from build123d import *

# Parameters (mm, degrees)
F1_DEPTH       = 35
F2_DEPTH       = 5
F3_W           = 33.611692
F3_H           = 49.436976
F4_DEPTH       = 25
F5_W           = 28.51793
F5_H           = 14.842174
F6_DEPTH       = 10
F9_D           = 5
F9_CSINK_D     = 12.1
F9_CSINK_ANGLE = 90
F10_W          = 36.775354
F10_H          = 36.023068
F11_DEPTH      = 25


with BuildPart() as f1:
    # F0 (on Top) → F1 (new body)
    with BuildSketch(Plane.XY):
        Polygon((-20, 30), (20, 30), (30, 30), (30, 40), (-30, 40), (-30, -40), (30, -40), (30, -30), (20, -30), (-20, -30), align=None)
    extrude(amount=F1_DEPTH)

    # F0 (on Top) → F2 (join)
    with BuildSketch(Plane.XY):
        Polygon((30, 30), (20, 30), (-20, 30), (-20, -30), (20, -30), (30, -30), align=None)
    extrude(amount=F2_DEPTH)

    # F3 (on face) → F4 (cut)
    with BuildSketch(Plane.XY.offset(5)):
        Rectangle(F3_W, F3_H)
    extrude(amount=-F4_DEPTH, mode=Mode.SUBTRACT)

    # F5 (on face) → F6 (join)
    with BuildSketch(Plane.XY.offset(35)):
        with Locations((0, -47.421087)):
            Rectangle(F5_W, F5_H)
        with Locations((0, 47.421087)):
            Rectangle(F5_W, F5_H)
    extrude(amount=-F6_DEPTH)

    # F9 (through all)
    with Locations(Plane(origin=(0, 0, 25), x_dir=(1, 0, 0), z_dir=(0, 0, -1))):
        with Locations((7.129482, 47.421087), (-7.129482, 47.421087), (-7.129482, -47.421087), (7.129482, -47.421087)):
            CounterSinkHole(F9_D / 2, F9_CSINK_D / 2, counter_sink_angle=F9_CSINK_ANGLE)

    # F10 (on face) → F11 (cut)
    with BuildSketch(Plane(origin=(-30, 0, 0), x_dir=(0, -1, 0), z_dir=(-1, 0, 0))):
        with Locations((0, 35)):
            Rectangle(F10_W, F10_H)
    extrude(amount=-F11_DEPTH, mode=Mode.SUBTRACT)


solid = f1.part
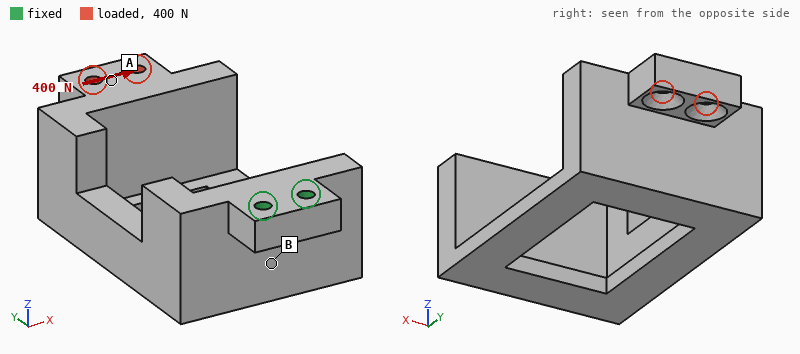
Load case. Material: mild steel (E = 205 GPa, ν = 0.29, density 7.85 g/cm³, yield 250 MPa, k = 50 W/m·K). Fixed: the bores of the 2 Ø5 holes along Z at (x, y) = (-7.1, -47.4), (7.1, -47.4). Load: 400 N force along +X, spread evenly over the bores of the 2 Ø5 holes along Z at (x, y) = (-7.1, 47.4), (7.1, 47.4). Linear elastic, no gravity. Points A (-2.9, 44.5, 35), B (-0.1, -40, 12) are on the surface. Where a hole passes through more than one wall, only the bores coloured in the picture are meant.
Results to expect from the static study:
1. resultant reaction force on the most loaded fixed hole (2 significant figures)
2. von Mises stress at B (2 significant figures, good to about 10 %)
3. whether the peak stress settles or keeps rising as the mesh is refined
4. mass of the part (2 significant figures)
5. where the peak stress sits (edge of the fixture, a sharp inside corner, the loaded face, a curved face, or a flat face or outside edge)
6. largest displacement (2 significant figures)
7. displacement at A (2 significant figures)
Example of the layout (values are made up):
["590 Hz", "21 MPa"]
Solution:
["2.1 kN", "28 MPa", "keeps rising", "550 g", "edge of the fixture", "0.13 mm", "0.12 mm"]
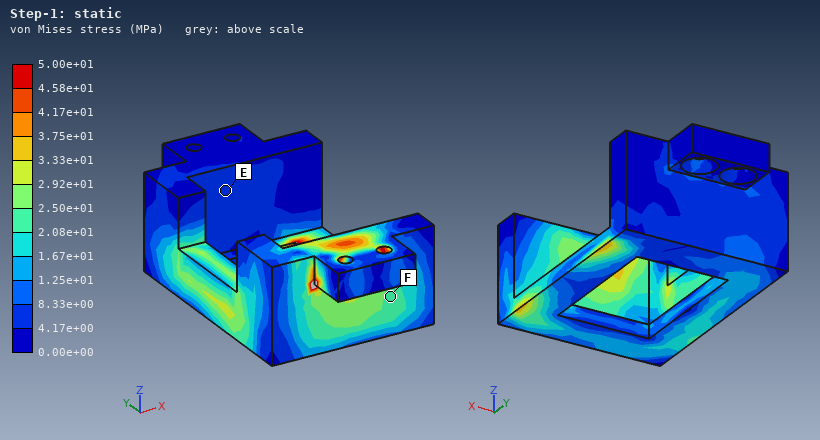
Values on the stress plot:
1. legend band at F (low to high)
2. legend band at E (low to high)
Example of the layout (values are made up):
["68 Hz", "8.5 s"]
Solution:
["2.08e+01 to 2.50e+01 MPa", "4.17e+00 to 8.33e+00 MPa"]
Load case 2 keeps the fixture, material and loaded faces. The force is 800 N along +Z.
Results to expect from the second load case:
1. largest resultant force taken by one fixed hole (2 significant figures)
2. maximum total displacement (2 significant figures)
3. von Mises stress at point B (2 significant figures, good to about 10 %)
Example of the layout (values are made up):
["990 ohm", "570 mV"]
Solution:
["700 N", "0.57 mm", "38 MPa"]
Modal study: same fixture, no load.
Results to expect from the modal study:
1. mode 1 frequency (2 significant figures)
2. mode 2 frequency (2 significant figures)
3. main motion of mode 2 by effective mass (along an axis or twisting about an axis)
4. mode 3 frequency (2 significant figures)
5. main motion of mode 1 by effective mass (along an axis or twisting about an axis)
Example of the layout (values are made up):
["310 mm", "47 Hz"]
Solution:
["470 Hz", "730 Hz", "along X", "1500 Hz", "along Z"]
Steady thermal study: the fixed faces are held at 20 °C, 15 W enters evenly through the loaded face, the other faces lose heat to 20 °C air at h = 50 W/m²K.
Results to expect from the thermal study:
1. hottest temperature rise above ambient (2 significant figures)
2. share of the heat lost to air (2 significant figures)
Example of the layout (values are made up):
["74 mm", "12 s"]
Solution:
["42 K", "88 %"]
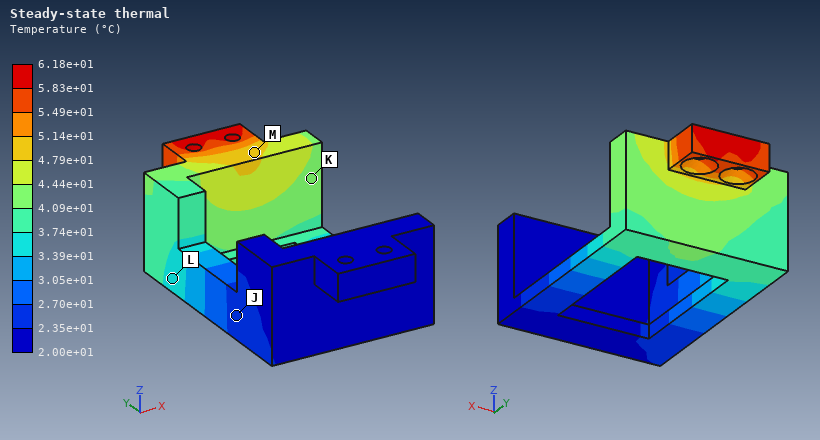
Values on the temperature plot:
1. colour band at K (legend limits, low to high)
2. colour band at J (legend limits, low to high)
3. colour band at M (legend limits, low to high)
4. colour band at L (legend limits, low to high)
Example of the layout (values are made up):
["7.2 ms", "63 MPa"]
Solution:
["4.09e+01 to 4.44e+01 °C", "2.35e+01 to 2.70e+01 °C", "4.79e+01 to 5.14e+01 °C", "3.39e+01 to 3.74e+01 °C"]
